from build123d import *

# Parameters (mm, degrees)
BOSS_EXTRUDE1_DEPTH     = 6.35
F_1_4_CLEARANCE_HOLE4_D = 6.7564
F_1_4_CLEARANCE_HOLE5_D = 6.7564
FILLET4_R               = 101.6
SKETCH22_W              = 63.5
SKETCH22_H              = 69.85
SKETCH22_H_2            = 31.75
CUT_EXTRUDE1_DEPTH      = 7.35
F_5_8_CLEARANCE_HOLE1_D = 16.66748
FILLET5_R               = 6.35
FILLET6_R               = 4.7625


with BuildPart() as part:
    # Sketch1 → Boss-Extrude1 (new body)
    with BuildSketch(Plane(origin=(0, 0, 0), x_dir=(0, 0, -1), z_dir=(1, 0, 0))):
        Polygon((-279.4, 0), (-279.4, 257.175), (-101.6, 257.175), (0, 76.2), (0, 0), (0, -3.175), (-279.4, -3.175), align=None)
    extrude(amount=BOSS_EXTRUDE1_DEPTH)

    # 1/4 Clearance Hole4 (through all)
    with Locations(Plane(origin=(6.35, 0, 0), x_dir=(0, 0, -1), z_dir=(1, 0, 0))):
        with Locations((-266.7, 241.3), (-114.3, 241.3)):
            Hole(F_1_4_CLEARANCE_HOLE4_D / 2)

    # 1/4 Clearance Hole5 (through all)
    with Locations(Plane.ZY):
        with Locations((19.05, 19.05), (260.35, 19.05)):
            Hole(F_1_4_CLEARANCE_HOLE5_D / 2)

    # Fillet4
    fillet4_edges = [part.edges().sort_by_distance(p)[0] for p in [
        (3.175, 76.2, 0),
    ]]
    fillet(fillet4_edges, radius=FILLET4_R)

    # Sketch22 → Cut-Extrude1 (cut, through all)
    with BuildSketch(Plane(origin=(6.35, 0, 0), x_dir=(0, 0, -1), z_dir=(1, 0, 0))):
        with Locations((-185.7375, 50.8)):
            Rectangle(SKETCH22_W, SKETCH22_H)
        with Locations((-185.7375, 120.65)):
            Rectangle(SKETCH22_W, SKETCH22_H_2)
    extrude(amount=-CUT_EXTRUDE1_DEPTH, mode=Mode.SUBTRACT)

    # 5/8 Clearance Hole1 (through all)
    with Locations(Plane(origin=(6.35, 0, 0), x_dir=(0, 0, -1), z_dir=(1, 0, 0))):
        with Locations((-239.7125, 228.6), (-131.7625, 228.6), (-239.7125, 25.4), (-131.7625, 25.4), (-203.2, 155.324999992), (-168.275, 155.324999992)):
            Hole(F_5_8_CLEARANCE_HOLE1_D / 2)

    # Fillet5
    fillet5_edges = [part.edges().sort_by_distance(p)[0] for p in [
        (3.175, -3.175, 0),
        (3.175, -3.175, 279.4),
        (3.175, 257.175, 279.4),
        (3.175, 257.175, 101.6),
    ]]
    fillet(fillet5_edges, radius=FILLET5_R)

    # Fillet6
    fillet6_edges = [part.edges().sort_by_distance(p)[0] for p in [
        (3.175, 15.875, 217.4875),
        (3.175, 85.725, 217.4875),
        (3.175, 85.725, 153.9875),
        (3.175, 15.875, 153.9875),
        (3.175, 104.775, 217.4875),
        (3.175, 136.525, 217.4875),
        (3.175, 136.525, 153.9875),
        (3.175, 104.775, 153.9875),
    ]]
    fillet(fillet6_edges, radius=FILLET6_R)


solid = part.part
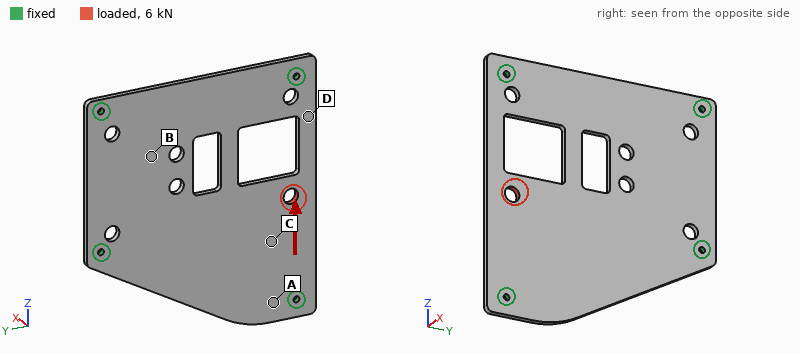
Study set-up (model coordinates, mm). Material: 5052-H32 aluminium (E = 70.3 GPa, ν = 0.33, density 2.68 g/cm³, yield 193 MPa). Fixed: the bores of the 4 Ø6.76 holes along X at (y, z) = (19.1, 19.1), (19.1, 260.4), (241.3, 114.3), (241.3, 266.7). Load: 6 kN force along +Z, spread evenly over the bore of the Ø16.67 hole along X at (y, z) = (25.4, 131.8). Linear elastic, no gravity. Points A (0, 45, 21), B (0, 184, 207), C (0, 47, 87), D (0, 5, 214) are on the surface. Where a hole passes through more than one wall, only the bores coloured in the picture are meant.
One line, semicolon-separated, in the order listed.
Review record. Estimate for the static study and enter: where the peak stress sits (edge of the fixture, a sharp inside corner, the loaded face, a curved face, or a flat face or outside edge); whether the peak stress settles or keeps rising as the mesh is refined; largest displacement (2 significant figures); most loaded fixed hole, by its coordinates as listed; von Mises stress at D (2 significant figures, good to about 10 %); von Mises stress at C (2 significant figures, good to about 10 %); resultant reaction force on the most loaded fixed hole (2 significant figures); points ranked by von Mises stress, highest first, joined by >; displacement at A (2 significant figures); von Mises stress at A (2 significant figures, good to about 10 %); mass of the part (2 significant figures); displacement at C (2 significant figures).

edge of the fixture; keeps rising; 28 µm; (19.1, 19.1); 10 MPa; 7.8 MPa; 3.7 kN; D > C > A > B; 7.4 µm; 4.5 MPa; 950 g; 13 µm
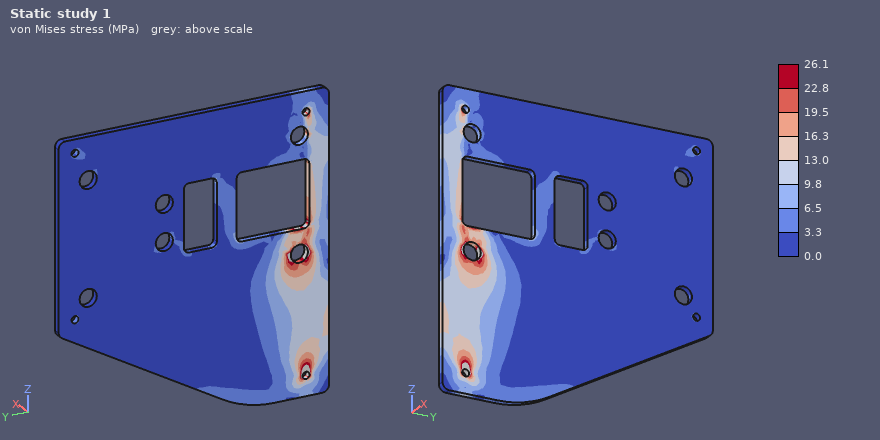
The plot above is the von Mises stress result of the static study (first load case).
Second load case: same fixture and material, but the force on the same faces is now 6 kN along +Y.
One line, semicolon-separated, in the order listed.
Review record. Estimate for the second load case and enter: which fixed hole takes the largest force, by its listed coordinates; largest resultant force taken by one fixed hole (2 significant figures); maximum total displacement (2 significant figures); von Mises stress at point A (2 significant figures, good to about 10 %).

(241.3, 114.3); 3.6 kN; 48 µm; 7.0 MPa
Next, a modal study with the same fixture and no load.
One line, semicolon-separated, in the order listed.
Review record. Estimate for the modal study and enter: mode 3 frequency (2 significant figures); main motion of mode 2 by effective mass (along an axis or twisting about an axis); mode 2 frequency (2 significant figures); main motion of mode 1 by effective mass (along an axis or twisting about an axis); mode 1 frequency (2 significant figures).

660 Hz; twisting about Y; 630 Hz; along X; 420 Hz
